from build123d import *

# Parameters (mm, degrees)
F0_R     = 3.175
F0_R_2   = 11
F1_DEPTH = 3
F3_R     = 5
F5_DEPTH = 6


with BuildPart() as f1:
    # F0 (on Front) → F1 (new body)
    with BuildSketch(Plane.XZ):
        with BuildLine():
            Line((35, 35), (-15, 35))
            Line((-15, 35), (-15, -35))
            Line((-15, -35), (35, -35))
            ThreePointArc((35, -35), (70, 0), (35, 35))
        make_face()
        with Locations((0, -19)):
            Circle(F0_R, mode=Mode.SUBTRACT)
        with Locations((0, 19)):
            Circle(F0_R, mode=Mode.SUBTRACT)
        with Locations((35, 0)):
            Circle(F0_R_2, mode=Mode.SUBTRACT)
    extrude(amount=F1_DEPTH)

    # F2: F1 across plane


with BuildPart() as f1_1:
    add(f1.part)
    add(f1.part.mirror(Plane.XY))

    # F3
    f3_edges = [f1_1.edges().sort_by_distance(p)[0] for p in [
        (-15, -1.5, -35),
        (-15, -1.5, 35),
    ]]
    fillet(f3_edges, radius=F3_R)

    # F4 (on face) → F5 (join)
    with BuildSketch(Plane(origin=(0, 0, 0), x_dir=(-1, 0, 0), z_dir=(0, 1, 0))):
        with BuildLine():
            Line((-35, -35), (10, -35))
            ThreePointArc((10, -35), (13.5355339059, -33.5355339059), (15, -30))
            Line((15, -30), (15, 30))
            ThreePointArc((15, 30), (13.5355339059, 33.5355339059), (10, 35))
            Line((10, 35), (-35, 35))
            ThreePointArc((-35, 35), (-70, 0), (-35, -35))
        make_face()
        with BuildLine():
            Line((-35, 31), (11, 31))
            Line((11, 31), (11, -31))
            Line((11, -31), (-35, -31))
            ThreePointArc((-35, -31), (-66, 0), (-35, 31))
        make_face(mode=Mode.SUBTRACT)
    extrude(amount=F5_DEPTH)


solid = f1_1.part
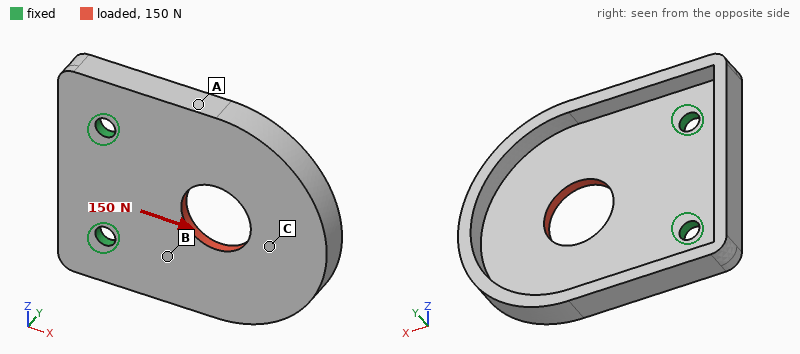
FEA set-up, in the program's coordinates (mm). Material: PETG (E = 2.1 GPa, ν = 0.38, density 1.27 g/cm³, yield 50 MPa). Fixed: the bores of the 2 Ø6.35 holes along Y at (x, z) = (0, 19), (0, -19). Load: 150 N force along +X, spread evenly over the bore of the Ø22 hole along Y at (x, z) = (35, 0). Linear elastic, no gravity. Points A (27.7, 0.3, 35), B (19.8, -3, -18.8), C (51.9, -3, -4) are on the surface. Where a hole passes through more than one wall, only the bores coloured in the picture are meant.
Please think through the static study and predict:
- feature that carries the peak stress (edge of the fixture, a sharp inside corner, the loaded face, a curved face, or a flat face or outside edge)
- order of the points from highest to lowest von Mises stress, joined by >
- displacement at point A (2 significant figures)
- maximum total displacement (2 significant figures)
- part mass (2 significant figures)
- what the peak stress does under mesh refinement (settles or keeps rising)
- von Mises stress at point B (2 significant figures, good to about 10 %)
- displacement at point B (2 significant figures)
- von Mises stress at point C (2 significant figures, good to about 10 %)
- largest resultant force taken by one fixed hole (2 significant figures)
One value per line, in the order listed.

edge of the fixture
B > C > A
16 µm
45 µm
27 g
keeps rising
0.99 MPa
11 µm
0.60 MPa
76 N
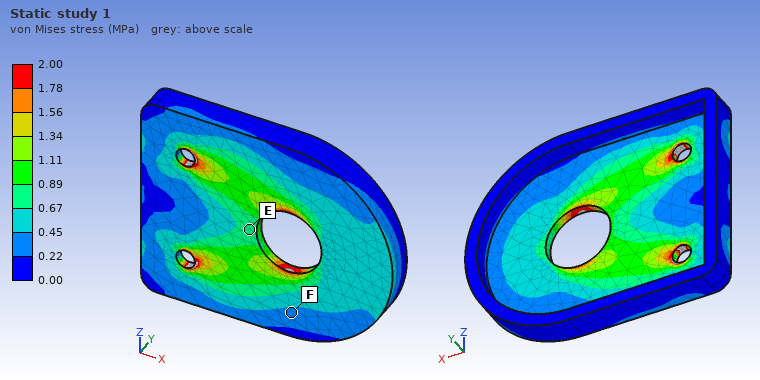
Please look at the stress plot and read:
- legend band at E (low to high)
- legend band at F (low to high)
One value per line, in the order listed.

0.67 to 0.89 MPa
0.22 to 0.45 MPa
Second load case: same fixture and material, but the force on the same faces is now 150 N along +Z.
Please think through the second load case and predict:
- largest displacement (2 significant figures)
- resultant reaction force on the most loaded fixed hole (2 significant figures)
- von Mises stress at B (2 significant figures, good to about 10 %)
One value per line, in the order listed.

0.13 mm
140 N
1.2 MPa
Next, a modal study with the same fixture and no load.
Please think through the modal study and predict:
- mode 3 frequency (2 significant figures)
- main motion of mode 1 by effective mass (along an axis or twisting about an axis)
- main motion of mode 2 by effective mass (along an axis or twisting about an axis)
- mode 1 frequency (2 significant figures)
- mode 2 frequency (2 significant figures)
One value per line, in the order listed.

1100 Hz
along Y
twisting about X
210 Hz
460 Hz
